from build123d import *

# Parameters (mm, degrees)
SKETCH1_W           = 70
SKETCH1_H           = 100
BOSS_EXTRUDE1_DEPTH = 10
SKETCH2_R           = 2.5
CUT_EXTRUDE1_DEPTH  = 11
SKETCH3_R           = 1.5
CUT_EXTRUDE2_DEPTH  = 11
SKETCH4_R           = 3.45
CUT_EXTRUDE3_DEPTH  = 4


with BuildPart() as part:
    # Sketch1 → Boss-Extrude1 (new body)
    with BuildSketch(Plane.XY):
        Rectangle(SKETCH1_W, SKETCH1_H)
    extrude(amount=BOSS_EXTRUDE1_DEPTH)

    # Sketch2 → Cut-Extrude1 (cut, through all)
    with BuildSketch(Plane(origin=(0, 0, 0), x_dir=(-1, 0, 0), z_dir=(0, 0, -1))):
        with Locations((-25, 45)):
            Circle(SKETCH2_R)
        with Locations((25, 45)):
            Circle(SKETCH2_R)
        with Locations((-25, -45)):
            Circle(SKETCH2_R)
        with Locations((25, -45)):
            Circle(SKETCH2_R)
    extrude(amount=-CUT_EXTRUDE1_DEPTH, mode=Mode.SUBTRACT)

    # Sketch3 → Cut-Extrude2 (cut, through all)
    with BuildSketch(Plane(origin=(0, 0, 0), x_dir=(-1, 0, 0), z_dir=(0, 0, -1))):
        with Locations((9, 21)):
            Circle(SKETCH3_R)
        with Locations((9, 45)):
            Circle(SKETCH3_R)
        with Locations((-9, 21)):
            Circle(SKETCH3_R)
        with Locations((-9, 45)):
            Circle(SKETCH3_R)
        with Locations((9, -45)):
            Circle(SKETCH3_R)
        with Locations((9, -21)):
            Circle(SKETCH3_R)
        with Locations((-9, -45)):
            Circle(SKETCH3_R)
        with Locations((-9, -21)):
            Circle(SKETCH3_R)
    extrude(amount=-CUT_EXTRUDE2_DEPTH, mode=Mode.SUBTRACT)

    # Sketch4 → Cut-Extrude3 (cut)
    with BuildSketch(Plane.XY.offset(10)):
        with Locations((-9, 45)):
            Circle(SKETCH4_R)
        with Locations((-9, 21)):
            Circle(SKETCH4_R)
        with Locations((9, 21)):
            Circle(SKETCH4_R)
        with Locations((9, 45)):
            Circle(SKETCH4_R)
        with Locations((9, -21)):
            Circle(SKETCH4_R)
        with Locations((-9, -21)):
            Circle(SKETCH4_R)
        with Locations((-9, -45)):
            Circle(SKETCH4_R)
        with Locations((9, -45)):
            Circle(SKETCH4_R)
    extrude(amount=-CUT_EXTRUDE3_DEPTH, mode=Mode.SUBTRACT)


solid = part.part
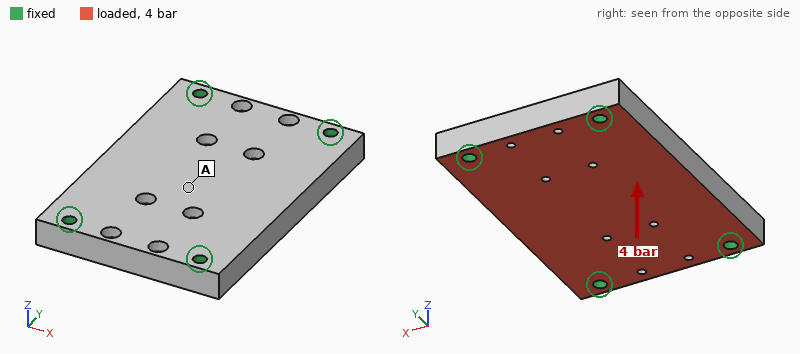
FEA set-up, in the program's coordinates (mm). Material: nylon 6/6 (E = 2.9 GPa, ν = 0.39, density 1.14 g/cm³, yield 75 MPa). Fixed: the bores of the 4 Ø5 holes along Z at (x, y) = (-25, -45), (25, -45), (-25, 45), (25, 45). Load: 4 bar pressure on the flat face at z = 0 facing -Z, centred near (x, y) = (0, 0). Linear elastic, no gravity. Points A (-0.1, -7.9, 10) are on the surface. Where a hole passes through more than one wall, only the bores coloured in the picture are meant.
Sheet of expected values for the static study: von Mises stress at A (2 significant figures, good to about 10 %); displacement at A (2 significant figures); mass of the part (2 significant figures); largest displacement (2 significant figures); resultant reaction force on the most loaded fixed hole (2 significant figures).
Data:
7.7 MPa
0.42 mm
77 g
0.45 mm
690 N
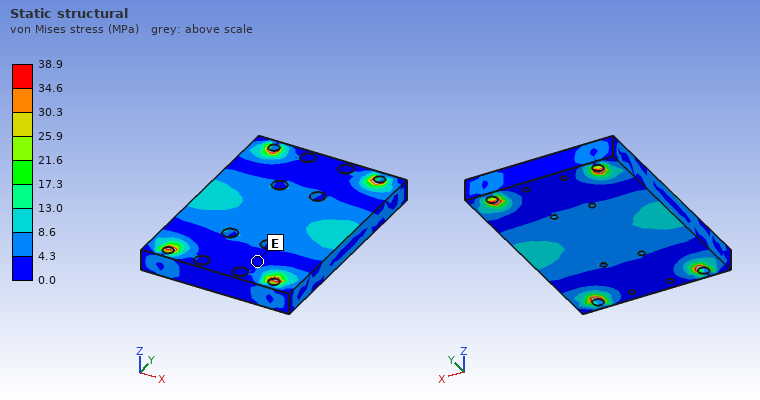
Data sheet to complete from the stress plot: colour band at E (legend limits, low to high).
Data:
0.0 to 4.3 MPa
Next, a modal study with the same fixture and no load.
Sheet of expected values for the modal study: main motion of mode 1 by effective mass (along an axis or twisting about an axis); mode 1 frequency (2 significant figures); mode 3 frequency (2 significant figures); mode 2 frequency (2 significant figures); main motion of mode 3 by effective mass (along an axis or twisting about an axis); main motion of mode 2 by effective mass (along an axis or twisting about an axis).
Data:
along Z
1600 Hz
4000 Hz
2300 Hz
twisting about X
twisting about Y
